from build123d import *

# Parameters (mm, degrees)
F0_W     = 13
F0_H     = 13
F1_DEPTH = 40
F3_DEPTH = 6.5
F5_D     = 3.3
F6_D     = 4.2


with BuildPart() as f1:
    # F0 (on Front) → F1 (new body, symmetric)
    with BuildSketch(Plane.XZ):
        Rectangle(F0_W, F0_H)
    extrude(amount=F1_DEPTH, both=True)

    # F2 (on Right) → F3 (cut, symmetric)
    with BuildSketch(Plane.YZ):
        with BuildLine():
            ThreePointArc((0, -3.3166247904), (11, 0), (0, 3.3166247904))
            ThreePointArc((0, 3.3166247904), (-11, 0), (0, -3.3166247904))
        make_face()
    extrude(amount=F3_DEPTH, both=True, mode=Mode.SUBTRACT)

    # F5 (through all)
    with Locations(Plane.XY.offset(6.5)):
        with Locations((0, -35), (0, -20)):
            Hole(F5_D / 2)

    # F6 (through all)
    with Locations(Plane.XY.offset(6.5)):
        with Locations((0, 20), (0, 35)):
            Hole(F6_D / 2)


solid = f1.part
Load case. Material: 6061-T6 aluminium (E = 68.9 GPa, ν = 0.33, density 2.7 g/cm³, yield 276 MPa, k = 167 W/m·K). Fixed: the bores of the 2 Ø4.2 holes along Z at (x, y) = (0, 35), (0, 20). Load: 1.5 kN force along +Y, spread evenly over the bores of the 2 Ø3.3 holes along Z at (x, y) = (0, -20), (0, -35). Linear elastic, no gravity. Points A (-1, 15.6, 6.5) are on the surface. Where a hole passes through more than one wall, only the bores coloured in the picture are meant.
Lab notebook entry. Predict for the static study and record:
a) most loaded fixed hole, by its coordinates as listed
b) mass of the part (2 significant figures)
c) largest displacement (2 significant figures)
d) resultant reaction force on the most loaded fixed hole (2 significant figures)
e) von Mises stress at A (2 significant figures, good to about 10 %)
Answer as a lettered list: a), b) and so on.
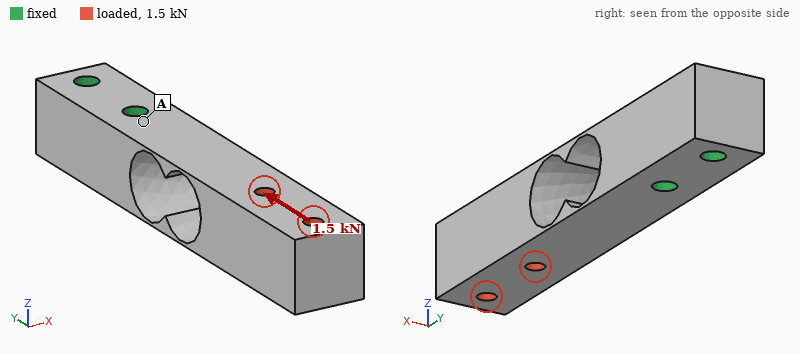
a) (0, 20)
b) 27 g
c) 32 µm
d) 1.4 kN
e) 25 MPa
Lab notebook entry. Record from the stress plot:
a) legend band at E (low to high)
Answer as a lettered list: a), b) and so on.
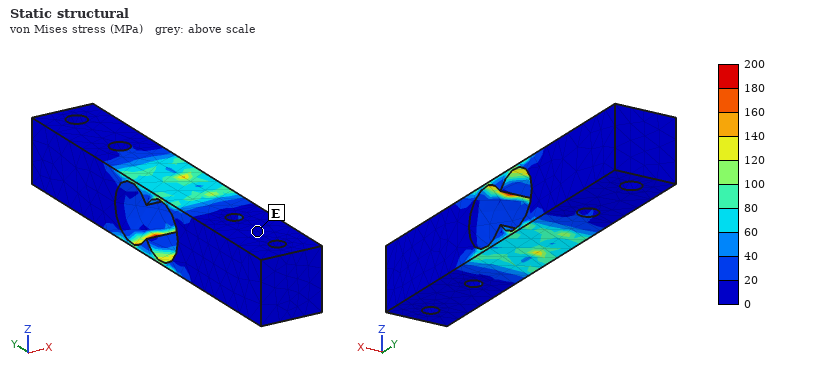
a) 0 to 20 MPa
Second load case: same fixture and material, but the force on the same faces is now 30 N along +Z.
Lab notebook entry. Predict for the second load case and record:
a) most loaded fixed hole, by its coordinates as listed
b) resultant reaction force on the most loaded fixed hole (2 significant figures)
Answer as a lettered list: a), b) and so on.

a) (0, 20)
b) 42 N
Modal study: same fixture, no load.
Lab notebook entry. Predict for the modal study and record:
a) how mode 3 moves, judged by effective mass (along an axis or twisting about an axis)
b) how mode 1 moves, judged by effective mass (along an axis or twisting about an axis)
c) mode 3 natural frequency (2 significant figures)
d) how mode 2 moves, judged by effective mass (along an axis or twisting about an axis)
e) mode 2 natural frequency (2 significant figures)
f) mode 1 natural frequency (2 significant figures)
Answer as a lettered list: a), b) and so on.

a) twisting about Y
b) along Z
c) 4800 Hz
d) along X
e) 1300 Hz
f) 580 Hz
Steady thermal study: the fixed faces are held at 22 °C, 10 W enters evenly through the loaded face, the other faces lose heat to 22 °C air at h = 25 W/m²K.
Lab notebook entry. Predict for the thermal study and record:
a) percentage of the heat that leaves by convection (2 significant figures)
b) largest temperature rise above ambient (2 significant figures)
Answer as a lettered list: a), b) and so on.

a) 27 %
b) 48 K
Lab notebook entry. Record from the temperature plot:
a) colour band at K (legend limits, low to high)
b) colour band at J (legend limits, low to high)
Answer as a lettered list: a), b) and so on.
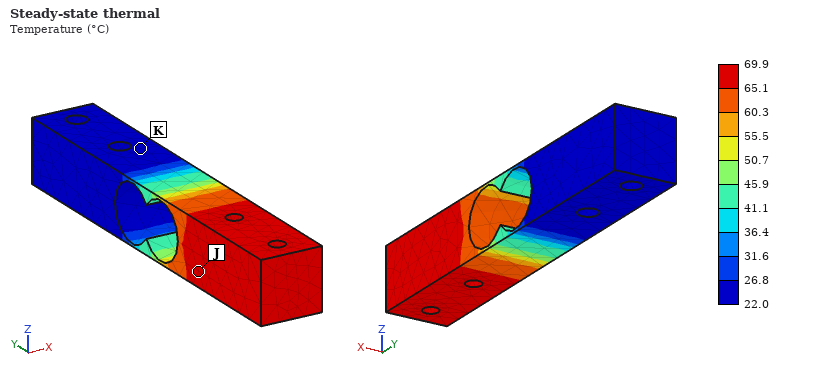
a) 22.0 to 26.8 °C
b) 65.1 to 69.9 °C
